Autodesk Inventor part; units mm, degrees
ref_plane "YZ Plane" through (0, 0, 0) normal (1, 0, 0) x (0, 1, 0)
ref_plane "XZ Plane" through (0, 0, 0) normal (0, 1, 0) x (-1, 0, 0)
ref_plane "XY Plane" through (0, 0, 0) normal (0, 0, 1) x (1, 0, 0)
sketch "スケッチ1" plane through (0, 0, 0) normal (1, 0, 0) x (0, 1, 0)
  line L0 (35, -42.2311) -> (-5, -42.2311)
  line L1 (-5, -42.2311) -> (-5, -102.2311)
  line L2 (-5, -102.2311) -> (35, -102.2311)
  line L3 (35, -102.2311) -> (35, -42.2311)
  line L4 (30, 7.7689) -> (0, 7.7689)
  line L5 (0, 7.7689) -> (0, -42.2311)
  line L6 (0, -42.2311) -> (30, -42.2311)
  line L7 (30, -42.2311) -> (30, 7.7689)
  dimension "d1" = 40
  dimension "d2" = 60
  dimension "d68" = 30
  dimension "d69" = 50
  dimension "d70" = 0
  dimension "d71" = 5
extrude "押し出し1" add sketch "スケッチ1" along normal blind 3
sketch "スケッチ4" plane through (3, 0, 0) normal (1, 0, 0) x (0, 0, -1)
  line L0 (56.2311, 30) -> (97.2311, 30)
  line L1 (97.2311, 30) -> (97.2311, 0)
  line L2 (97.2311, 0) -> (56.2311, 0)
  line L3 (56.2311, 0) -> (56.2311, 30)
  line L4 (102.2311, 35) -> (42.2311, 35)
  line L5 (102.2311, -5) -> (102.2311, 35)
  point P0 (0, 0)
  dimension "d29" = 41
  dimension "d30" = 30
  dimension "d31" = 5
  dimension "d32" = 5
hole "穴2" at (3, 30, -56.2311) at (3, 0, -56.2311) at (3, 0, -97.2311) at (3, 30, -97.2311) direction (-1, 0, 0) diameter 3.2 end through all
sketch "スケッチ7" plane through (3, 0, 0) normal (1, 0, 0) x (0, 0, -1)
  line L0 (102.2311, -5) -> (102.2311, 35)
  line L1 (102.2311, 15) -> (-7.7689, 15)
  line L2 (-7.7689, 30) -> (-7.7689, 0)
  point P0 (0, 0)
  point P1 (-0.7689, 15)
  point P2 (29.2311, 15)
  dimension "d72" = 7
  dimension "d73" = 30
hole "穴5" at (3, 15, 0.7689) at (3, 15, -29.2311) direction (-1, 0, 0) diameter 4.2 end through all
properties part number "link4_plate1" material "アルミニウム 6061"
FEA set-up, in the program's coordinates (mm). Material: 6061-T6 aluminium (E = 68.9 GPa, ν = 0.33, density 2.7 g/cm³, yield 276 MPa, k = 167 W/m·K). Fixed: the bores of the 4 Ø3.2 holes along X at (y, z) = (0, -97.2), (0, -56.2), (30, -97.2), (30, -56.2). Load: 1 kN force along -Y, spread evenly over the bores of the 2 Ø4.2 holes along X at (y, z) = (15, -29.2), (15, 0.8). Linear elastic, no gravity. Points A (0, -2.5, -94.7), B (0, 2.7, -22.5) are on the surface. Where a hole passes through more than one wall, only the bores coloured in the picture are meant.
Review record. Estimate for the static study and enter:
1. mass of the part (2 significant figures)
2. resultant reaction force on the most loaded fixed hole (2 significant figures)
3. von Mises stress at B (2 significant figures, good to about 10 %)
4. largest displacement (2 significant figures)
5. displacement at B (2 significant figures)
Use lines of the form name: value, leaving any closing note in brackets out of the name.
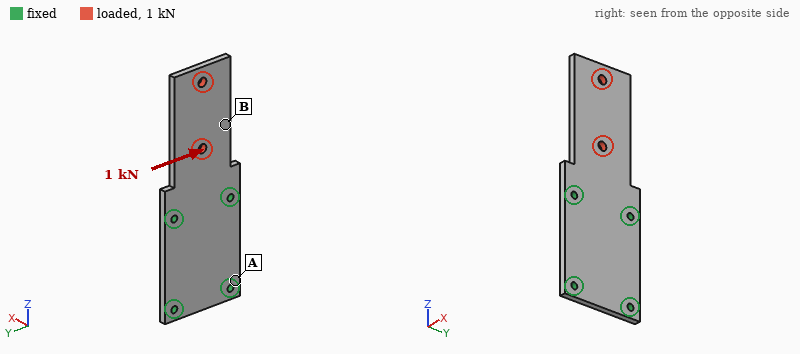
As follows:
mass of the part: 31 g
resultant reaction force on the most loaded fixed hole: 1.4 kN
von Mises stress at B: 20 MPa
largest displacement: 98 µm
displacement at B: 43 µm
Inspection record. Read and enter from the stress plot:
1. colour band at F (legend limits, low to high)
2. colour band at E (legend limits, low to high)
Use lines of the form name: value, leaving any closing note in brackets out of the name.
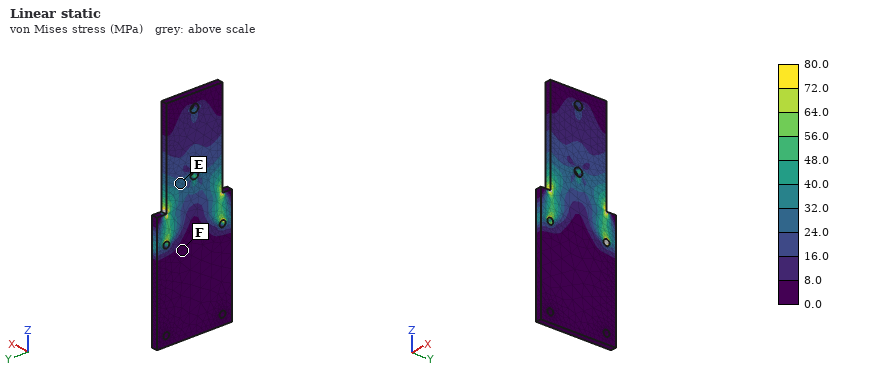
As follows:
colour band at F: 0.0 to 8.0 MPa
colour band at E: 24.0 to 32.0 MPa
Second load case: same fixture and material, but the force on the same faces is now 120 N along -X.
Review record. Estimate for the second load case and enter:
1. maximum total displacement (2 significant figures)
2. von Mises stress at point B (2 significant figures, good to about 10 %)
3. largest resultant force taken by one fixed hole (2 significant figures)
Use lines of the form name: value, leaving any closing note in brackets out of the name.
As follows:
maximum total displacement: 1.1 mm
von Mises stress at point B: 33 MPa
largest resultant force taken by one fixed hole: 74 N
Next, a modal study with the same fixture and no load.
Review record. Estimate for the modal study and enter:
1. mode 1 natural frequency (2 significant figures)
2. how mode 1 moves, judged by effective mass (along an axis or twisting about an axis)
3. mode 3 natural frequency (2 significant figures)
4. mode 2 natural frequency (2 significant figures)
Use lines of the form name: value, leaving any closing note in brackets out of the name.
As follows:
mode 1 natural frequency: 630 Hz
how mode 1 moves, judged by effective mass: along X
mode 3 natural frequency: 3700 Hz
mode 2 natural frequency: 2800 Hz
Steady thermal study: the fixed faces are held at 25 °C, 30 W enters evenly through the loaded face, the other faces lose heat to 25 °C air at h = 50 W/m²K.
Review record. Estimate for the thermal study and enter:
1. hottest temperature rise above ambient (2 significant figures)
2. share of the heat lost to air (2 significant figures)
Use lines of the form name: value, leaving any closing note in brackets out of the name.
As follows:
hottest temperature rise above ambient: 69 K
share of the heat lost to air: 29 %
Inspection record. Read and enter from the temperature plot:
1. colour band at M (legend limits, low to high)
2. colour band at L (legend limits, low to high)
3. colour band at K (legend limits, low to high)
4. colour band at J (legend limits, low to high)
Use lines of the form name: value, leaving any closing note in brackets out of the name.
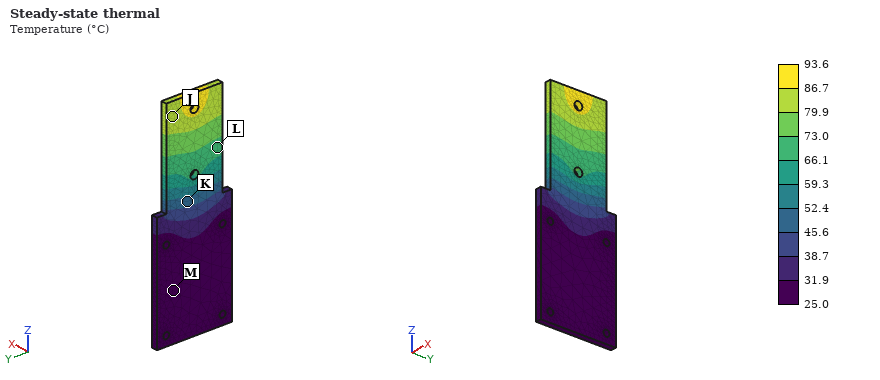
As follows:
colour band at M: 25.0 to 31.9 °C
colour band at L: 66.1 to 73.0 °C
colour band at K: 45.6 to 52.4 °C
colour band at J: 79.9 to 86.7 °C
